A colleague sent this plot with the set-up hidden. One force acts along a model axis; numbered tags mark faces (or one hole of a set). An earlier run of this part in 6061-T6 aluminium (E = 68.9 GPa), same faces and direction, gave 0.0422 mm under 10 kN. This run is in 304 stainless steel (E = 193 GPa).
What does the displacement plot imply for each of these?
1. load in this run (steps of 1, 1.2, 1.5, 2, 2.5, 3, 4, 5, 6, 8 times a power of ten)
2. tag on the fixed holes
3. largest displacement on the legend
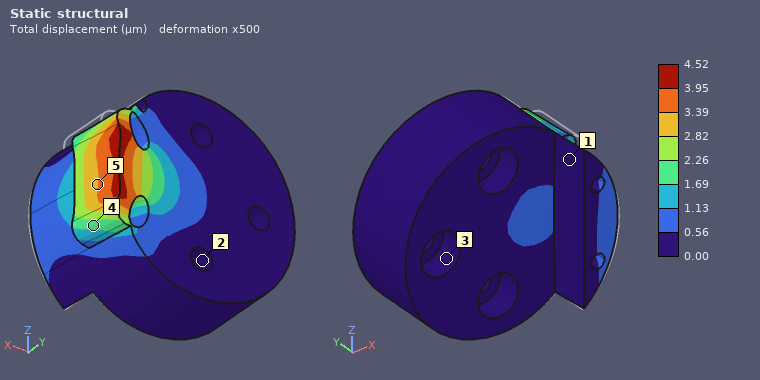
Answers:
3 kN
2
4.52 µm
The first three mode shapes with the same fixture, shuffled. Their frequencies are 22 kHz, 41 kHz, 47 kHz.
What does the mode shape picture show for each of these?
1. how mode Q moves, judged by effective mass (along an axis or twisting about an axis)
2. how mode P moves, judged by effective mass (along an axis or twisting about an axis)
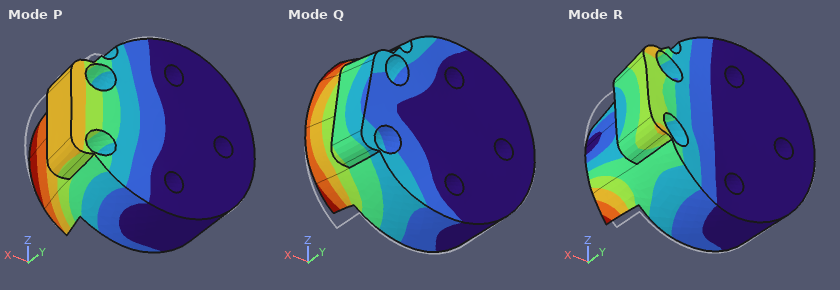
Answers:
along Z
along Y
